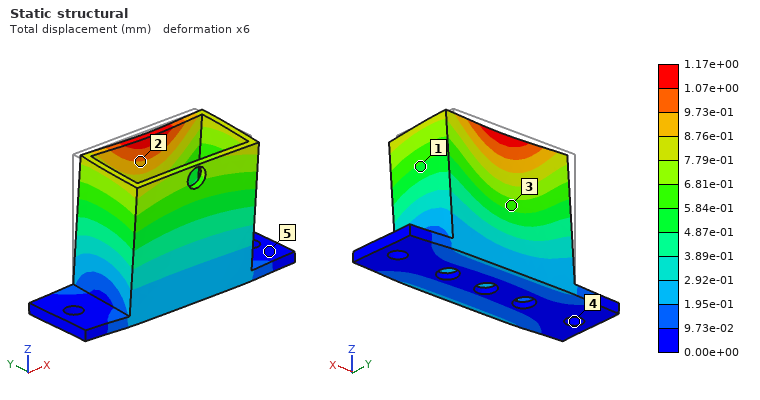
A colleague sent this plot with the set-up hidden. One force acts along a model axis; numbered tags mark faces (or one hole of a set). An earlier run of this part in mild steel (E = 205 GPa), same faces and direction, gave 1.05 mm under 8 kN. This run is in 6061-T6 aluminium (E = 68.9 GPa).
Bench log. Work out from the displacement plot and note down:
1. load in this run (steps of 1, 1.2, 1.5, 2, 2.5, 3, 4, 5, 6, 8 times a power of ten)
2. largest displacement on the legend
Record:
3 kN
1.17e+00 mm
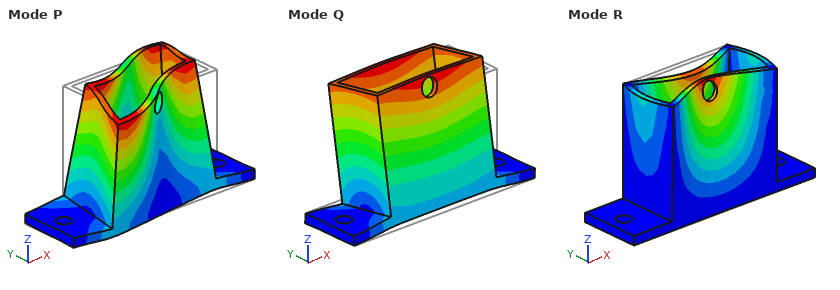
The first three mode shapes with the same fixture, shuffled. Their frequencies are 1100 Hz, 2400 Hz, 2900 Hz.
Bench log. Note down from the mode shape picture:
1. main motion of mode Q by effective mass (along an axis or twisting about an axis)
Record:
along Y
